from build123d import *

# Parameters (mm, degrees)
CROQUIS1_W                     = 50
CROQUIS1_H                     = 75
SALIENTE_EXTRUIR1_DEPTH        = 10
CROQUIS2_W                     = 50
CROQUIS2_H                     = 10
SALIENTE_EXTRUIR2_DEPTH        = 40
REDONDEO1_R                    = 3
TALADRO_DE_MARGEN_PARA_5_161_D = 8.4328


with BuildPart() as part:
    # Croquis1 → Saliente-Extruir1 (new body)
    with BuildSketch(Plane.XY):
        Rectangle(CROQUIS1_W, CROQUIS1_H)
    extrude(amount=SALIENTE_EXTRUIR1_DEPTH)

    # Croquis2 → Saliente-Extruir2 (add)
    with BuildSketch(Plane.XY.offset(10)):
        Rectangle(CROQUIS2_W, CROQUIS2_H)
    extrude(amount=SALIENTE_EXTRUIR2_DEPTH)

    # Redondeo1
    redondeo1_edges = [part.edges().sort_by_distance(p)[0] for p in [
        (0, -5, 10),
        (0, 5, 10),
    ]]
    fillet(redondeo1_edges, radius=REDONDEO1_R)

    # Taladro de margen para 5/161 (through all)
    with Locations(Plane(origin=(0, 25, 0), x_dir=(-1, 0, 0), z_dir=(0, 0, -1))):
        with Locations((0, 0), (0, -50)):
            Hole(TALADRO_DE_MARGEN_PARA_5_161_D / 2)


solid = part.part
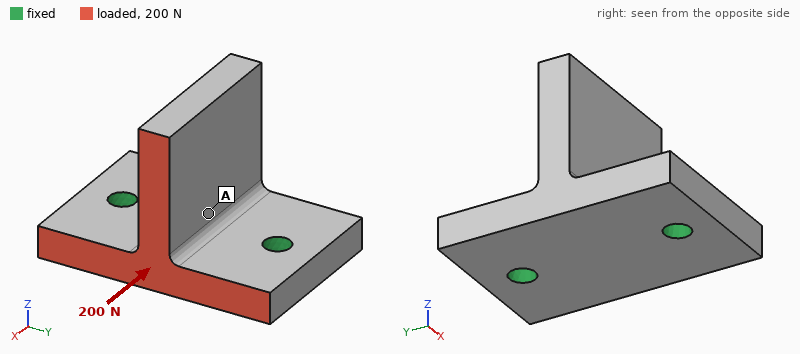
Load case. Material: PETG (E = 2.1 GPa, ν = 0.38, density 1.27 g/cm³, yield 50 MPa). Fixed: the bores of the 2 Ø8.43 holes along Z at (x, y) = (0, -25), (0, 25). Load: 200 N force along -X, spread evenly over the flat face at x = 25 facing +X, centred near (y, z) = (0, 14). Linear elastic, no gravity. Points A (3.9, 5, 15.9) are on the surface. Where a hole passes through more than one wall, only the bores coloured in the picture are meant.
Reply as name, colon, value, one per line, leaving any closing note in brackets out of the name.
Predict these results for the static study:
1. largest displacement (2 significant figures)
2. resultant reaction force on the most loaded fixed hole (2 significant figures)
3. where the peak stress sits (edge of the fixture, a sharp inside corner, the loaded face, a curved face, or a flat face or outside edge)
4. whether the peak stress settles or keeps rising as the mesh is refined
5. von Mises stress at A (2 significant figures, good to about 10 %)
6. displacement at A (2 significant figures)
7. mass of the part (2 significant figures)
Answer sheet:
largest displacement: 80 µm
resultant reaction force on the most loaded fixed hole: 100 N
where the peak stress sits: edge of the fixture
whether the peak stress settles or keeps rising as the mesh is refined: keeps rising
von Mises stress at A: 0.35 MPa
displacement at A: 21 µm
mass of the part: 72 g
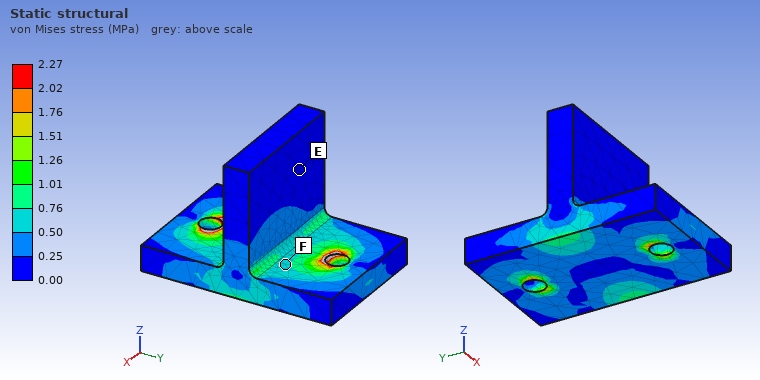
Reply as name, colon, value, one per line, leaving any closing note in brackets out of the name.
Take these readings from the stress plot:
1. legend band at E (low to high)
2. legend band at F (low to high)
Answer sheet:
legend band at E: 0.00 to 0.25 MPa
legend band at F: 0.50 to 0.76 MPa
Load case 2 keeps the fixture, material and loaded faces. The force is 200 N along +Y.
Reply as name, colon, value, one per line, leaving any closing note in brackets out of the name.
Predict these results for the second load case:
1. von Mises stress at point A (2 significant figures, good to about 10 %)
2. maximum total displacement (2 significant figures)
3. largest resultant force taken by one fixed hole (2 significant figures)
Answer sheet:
von Mises stress at point A: 1.5 MPa
maximum total displacement: 0.16 mm
largest resultant force taken by one fixed hole: 140 N
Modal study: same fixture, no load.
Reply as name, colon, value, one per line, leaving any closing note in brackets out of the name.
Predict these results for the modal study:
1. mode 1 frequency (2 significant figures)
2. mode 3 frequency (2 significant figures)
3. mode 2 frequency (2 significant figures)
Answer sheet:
mode 1 frequency: 1000 Hz
mode 3 frequency: 2100 Hz
mode 2 frequency: 1100 Hz
